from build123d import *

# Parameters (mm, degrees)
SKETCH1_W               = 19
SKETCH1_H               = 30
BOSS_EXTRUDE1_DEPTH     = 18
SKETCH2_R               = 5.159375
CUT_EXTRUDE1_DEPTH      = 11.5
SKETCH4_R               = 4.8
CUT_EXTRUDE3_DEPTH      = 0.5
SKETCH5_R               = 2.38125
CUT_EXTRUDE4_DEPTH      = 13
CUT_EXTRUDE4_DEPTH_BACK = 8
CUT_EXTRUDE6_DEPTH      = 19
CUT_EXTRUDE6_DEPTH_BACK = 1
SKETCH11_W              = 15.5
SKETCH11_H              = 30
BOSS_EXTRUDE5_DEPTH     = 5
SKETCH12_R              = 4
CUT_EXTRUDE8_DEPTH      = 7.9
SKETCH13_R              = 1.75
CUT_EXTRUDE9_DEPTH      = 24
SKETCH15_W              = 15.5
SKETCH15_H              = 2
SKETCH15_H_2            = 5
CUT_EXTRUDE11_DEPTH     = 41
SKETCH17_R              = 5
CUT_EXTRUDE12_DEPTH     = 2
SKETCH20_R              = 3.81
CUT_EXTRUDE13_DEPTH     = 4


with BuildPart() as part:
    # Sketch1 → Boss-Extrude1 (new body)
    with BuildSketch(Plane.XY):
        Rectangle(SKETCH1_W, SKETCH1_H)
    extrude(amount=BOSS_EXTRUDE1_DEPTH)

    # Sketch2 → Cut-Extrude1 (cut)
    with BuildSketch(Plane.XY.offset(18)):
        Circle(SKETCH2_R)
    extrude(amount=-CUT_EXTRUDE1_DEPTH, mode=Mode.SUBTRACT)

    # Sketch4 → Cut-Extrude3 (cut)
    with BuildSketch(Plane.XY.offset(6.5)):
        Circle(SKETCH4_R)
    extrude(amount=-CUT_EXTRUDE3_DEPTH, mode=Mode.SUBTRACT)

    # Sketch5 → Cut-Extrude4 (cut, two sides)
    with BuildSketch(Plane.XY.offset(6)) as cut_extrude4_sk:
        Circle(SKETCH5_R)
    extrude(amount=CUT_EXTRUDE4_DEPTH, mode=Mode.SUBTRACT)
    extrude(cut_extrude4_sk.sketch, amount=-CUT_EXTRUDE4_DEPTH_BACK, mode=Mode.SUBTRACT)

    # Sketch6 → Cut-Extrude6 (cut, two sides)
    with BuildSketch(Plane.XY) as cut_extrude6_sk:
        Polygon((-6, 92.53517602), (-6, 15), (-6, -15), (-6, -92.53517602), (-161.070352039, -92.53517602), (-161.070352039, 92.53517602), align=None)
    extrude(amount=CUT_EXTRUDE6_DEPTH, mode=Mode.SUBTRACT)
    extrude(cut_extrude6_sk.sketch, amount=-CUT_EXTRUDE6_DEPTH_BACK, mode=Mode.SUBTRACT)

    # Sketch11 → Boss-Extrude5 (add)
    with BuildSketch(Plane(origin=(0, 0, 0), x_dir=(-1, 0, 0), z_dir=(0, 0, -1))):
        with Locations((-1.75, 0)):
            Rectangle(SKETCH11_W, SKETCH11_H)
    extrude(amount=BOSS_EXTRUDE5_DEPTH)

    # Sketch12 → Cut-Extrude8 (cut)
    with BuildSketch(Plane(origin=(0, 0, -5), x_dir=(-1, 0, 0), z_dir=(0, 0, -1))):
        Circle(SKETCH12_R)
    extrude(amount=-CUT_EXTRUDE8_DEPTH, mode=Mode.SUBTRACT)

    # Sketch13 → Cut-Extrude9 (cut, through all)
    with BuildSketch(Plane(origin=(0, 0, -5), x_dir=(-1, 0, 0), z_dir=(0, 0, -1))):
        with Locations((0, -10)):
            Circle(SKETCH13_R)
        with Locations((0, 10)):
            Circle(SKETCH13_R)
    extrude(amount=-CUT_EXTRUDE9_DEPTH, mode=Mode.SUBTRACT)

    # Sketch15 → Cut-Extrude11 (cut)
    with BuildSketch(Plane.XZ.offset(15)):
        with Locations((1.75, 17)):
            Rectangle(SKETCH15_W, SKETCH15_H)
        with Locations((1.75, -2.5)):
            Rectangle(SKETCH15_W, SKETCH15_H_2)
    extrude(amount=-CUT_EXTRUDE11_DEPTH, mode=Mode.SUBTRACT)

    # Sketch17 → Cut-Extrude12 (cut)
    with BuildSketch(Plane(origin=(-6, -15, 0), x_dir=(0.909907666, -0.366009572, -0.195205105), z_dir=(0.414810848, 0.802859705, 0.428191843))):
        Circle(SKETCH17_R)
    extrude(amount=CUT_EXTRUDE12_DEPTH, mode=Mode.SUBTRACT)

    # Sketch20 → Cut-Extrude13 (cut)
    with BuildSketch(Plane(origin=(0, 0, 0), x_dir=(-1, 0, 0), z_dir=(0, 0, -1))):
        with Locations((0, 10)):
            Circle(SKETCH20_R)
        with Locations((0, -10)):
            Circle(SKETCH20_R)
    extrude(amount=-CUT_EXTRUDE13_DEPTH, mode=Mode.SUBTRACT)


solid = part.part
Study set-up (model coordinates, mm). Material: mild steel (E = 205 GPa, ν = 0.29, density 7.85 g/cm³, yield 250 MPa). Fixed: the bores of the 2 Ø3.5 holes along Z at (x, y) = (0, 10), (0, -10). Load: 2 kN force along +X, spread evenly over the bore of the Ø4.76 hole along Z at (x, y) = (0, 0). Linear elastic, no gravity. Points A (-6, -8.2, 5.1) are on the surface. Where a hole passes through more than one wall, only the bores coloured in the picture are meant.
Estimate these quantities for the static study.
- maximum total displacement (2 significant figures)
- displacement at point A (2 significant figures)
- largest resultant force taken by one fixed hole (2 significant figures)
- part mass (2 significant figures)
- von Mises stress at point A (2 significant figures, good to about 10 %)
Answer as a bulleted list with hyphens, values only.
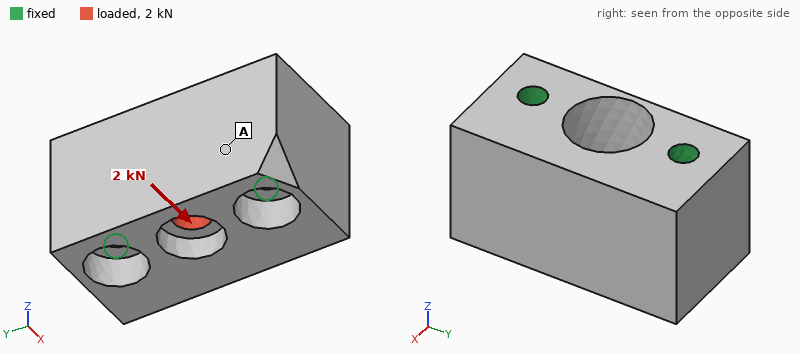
- 2.8 µm
- 0.73 µm
- 1.0 kN
- 46 g
- 14 MPa
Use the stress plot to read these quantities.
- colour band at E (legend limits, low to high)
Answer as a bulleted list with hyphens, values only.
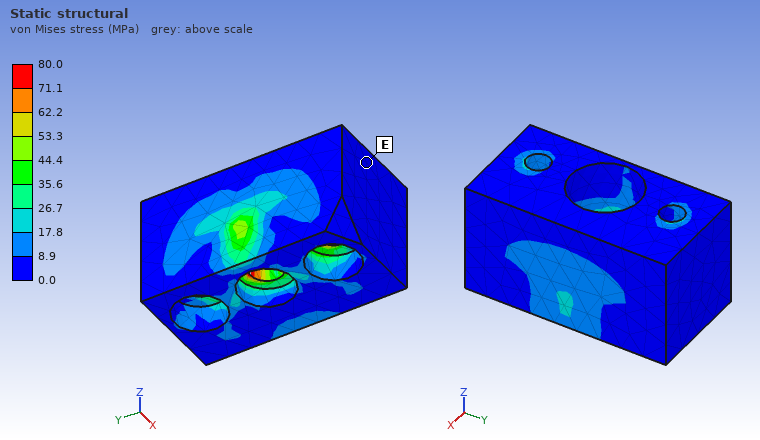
- 0.0 to 8.9 MPa
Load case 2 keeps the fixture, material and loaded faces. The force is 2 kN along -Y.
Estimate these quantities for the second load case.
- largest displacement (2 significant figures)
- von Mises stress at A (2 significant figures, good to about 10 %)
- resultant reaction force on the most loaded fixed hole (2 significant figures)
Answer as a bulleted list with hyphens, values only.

- 1.4 µm
- 7.2 MPa
- 1.0 kN
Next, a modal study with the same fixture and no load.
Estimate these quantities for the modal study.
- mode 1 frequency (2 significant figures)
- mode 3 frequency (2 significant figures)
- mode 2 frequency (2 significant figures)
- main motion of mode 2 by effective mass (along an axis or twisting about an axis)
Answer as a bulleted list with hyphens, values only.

- 41 kHz
- 55 kHz
- 51 kHz
- along Y
